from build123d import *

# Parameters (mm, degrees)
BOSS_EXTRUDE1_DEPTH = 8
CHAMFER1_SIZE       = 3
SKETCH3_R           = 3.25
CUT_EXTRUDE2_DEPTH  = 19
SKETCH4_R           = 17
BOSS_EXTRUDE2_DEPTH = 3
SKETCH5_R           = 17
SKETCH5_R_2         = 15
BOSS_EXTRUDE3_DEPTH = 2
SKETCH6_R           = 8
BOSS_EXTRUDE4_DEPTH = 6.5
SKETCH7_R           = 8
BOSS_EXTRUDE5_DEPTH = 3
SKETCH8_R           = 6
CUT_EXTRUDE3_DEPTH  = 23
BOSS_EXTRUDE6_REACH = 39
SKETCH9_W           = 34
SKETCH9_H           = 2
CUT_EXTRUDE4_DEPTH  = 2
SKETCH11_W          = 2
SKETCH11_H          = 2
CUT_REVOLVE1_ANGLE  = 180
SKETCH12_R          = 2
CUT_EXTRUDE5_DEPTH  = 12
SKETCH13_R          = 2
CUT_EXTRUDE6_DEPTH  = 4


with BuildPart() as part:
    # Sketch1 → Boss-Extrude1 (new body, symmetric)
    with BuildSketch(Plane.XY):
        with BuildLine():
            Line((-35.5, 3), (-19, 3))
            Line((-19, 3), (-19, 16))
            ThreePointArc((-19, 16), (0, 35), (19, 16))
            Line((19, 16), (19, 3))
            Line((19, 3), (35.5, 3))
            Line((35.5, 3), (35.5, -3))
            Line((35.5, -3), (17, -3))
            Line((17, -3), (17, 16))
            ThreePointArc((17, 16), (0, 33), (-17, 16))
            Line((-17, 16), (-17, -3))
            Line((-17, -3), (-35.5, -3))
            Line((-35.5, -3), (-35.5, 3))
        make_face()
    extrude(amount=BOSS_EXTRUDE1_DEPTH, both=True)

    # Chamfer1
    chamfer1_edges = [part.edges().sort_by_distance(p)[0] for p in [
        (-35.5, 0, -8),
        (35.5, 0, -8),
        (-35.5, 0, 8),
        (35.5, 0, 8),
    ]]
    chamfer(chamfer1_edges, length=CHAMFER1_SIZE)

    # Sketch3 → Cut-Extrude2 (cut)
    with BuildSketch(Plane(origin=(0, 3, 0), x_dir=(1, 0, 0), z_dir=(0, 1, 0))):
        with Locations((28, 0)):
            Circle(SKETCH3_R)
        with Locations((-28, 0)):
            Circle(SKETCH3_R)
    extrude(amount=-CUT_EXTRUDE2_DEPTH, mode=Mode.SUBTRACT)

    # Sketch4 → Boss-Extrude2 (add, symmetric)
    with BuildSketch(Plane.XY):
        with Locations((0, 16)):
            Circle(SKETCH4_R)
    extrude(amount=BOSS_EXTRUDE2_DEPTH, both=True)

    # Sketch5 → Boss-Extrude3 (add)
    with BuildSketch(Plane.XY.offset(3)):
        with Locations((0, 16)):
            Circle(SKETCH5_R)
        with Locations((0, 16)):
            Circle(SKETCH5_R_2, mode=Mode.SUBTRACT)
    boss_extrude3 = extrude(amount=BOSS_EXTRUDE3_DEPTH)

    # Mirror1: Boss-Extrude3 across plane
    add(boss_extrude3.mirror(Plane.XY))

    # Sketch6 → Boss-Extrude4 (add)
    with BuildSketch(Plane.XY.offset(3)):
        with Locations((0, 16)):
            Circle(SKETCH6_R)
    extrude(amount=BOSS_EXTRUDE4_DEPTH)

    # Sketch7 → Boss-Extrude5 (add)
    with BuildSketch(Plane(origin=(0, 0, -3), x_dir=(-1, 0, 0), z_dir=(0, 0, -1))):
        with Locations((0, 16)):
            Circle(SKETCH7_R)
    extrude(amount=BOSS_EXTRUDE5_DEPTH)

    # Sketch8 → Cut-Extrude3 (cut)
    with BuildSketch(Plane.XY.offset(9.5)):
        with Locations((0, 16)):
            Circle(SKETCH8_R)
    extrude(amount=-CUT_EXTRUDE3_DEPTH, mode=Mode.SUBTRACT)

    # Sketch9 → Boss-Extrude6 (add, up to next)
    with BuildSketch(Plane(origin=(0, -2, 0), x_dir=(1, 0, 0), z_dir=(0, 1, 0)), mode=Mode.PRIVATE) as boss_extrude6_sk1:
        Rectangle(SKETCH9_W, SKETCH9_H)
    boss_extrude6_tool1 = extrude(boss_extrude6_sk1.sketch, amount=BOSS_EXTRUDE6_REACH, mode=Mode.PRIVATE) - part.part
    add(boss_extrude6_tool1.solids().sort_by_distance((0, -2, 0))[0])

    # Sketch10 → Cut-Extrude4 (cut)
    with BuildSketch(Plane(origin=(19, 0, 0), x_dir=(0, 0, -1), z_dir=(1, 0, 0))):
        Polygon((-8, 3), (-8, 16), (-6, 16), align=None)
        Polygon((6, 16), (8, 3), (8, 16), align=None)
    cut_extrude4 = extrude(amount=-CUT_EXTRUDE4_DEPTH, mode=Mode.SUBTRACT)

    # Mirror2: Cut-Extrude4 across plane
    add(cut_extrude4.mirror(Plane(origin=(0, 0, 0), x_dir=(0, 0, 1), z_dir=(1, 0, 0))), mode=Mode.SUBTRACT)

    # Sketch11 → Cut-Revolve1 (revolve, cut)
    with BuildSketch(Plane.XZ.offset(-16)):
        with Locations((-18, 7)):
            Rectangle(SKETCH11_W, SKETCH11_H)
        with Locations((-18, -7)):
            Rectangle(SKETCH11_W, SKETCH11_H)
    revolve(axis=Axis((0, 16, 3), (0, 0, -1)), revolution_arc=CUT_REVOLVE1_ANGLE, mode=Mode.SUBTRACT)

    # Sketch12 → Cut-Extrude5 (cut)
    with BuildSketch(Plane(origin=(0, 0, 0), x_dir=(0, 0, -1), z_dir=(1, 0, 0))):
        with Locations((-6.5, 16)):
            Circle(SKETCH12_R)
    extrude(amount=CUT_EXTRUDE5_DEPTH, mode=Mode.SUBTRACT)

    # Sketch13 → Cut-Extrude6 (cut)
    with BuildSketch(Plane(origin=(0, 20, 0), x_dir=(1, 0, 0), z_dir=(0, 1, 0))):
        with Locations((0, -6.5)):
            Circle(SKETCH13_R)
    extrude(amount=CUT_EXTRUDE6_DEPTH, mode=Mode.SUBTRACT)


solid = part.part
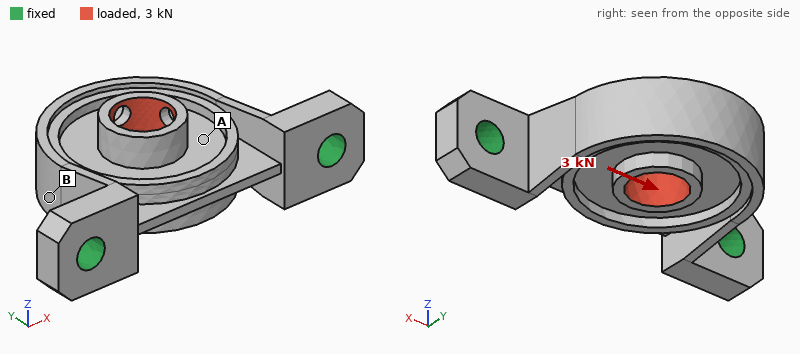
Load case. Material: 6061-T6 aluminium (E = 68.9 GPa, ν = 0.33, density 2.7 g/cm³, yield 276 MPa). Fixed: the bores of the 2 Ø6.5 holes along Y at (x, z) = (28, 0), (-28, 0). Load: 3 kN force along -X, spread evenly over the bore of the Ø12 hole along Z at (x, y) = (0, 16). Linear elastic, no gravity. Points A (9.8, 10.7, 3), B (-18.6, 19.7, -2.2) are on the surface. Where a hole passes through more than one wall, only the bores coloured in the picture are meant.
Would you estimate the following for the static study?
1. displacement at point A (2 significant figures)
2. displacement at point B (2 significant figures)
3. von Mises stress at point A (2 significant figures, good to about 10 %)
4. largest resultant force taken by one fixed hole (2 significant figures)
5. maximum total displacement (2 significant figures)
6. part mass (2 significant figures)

22 µm
34 µm
27 MPa
1.9 kN
47 µm
32 g
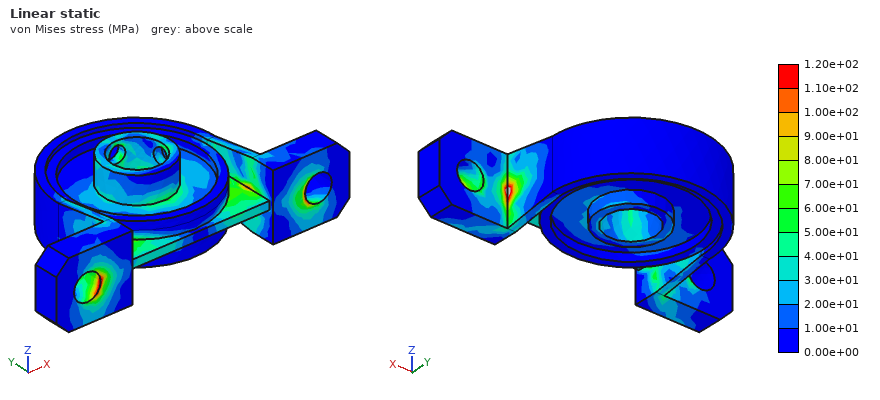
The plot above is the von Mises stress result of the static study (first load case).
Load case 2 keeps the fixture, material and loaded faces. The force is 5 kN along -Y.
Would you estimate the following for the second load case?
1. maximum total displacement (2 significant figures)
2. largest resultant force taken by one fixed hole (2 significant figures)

0.11 mm
2.7 kN
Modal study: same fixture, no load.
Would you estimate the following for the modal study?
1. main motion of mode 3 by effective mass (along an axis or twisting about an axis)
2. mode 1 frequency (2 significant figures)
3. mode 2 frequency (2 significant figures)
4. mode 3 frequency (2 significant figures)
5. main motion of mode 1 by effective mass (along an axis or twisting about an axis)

along X
3200 Hz
9200 Hz
9500 Hz
along Z
